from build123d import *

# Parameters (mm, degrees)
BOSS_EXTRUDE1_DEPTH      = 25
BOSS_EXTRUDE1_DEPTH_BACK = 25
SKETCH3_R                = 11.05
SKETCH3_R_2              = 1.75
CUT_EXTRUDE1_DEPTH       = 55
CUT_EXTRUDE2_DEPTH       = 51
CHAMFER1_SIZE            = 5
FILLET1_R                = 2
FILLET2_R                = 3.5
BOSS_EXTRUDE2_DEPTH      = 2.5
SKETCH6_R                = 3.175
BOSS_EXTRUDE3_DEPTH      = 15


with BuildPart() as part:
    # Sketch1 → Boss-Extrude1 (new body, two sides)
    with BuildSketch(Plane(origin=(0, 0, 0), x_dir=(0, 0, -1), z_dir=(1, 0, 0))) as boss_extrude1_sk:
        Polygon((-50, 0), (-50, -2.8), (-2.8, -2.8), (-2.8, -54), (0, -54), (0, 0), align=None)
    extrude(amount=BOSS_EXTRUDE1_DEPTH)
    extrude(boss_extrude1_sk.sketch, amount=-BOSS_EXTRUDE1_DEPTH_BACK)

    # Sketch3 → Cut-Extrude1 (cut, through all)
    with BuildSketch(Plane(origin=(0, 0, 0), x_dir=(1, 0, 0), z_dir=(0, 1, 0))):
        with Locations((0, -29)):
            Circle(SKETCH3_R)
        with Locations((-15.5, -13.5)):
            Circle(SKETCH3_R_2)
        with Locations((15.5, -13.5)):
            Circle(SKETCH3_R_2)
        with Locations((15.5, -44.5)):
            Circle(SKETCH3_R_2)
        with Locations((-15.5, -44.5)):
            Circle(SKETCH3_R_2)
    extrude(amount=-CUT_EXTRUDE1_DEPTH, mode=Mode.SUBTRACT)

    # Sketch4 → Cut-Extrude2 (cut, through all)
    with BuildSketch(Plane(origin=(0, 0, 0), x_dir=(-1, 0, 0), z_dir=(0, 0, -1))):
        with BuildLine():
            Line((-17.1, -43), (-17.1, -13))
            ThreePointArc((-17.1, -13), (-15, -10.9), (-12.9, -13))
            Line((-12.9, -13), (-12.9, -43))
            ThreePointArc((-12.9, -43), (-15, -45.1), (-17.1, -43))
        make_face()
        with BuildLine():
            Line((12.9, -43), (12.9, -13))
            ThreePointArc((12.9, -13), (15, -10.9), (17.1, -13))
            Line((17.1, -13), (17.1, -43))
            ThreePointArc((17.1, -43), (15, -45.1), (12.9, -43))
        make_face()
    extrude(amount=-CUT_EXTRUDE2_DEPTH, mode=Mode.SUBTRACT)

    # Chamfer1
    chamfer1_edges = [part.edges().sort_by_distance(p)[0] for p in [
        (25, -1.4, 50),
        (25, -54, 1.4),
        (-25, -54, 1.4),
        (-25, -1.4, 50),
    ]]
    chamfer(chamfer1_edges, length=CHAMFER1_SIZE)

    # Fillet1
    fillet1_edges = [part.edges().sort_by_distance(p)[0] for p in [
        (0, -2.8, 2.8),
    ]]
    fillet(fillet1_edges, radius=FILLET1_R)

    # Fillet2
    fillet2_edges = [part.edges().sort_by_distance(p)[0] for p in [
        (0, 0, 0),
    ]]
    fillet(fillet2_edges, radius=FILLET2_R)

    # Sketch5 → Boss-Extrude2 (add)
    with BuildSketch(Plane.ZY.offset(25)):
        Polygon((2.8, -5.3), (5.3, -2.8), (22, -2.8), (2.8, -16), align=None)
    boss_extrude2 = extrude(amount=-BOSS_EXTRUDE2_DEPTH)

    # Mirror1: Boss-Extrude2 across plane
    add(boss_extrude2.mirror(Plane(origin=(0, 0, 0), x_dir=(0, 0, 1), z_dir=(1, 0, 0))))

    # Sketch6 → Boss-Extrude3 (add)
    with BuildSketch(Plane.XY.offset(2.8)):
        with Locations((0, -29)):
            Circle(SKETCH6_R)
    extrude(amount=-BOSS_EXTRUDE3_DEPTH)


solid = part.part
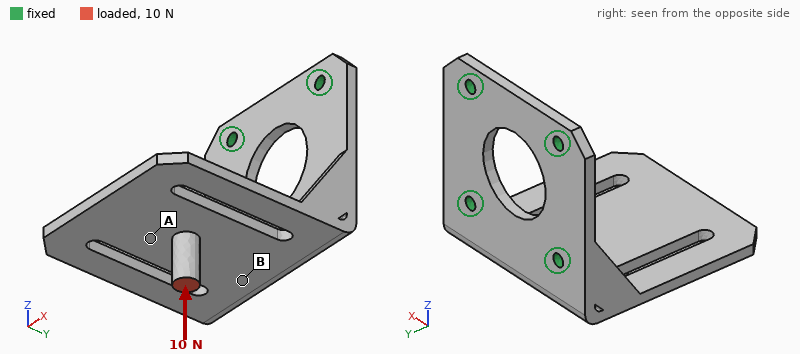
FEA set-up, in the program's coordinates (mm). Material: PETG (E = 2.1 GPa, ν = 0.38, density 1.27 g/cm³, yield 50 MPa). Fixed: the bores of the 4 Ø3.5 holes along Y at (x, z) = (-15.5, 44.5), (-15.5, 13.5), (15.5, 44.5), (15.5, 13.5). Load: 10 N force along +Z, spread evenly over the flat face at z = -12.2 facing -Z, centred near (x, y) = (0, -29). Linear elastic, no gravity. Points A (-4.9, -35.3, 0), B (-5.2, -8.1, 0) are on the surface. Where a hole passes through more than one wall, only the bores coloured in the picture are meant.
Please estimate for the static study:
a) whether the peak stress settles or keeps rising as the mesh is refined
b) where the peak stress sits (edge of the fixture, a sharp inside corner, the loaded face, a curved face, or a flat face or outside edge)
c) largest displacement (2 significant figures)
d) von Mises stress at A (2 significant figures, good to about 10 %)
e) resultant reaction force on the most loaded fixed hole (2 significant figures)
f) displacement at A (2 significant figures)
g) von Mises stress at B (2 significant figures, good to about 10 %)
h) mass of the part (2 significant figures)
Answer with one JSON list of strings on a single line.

["keeps rising", "edge of the fixture", "0.98 mm", "0.68 MPa", "6.2 N", "0.59 mm", "2.2 MPa", "16 g"]
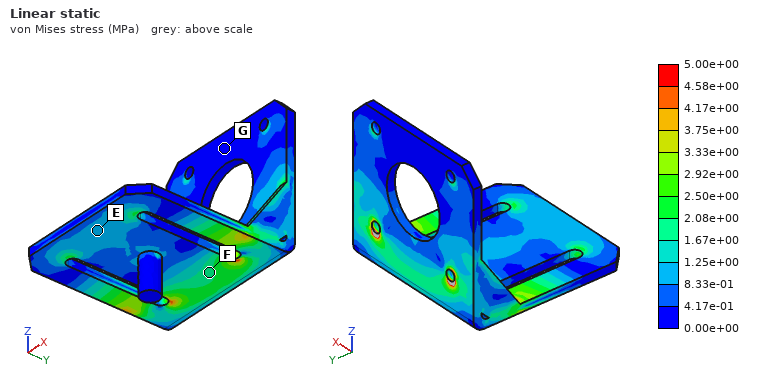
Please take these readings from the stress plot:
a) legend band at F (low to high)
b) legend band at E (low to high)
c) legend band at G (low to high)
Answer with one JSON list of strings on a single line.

["1.67e+00 to 2.08e+00 MPa", "8.33e-01 to 1.25e+00 MPa", "0.00e+00 to 4.17e-01 MPa"]
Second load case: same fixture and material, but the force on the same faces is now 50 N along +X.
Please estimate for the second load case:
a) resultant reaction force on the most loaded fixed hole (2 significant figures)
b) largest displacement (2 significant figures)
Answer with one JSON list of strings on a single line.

["56 N", "1.1 mm"]
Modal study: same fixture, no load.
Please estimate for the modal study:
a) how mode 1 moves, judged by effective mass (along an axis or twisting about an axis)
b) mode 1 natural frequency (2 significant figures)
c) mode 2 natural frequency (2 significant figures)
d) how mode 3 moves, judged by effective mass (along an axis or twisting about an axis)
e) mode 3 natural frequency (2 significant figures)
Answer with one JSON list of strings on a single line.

["along Z", "210 Hz", "520 Hz", "along X", "760 Hz"]
